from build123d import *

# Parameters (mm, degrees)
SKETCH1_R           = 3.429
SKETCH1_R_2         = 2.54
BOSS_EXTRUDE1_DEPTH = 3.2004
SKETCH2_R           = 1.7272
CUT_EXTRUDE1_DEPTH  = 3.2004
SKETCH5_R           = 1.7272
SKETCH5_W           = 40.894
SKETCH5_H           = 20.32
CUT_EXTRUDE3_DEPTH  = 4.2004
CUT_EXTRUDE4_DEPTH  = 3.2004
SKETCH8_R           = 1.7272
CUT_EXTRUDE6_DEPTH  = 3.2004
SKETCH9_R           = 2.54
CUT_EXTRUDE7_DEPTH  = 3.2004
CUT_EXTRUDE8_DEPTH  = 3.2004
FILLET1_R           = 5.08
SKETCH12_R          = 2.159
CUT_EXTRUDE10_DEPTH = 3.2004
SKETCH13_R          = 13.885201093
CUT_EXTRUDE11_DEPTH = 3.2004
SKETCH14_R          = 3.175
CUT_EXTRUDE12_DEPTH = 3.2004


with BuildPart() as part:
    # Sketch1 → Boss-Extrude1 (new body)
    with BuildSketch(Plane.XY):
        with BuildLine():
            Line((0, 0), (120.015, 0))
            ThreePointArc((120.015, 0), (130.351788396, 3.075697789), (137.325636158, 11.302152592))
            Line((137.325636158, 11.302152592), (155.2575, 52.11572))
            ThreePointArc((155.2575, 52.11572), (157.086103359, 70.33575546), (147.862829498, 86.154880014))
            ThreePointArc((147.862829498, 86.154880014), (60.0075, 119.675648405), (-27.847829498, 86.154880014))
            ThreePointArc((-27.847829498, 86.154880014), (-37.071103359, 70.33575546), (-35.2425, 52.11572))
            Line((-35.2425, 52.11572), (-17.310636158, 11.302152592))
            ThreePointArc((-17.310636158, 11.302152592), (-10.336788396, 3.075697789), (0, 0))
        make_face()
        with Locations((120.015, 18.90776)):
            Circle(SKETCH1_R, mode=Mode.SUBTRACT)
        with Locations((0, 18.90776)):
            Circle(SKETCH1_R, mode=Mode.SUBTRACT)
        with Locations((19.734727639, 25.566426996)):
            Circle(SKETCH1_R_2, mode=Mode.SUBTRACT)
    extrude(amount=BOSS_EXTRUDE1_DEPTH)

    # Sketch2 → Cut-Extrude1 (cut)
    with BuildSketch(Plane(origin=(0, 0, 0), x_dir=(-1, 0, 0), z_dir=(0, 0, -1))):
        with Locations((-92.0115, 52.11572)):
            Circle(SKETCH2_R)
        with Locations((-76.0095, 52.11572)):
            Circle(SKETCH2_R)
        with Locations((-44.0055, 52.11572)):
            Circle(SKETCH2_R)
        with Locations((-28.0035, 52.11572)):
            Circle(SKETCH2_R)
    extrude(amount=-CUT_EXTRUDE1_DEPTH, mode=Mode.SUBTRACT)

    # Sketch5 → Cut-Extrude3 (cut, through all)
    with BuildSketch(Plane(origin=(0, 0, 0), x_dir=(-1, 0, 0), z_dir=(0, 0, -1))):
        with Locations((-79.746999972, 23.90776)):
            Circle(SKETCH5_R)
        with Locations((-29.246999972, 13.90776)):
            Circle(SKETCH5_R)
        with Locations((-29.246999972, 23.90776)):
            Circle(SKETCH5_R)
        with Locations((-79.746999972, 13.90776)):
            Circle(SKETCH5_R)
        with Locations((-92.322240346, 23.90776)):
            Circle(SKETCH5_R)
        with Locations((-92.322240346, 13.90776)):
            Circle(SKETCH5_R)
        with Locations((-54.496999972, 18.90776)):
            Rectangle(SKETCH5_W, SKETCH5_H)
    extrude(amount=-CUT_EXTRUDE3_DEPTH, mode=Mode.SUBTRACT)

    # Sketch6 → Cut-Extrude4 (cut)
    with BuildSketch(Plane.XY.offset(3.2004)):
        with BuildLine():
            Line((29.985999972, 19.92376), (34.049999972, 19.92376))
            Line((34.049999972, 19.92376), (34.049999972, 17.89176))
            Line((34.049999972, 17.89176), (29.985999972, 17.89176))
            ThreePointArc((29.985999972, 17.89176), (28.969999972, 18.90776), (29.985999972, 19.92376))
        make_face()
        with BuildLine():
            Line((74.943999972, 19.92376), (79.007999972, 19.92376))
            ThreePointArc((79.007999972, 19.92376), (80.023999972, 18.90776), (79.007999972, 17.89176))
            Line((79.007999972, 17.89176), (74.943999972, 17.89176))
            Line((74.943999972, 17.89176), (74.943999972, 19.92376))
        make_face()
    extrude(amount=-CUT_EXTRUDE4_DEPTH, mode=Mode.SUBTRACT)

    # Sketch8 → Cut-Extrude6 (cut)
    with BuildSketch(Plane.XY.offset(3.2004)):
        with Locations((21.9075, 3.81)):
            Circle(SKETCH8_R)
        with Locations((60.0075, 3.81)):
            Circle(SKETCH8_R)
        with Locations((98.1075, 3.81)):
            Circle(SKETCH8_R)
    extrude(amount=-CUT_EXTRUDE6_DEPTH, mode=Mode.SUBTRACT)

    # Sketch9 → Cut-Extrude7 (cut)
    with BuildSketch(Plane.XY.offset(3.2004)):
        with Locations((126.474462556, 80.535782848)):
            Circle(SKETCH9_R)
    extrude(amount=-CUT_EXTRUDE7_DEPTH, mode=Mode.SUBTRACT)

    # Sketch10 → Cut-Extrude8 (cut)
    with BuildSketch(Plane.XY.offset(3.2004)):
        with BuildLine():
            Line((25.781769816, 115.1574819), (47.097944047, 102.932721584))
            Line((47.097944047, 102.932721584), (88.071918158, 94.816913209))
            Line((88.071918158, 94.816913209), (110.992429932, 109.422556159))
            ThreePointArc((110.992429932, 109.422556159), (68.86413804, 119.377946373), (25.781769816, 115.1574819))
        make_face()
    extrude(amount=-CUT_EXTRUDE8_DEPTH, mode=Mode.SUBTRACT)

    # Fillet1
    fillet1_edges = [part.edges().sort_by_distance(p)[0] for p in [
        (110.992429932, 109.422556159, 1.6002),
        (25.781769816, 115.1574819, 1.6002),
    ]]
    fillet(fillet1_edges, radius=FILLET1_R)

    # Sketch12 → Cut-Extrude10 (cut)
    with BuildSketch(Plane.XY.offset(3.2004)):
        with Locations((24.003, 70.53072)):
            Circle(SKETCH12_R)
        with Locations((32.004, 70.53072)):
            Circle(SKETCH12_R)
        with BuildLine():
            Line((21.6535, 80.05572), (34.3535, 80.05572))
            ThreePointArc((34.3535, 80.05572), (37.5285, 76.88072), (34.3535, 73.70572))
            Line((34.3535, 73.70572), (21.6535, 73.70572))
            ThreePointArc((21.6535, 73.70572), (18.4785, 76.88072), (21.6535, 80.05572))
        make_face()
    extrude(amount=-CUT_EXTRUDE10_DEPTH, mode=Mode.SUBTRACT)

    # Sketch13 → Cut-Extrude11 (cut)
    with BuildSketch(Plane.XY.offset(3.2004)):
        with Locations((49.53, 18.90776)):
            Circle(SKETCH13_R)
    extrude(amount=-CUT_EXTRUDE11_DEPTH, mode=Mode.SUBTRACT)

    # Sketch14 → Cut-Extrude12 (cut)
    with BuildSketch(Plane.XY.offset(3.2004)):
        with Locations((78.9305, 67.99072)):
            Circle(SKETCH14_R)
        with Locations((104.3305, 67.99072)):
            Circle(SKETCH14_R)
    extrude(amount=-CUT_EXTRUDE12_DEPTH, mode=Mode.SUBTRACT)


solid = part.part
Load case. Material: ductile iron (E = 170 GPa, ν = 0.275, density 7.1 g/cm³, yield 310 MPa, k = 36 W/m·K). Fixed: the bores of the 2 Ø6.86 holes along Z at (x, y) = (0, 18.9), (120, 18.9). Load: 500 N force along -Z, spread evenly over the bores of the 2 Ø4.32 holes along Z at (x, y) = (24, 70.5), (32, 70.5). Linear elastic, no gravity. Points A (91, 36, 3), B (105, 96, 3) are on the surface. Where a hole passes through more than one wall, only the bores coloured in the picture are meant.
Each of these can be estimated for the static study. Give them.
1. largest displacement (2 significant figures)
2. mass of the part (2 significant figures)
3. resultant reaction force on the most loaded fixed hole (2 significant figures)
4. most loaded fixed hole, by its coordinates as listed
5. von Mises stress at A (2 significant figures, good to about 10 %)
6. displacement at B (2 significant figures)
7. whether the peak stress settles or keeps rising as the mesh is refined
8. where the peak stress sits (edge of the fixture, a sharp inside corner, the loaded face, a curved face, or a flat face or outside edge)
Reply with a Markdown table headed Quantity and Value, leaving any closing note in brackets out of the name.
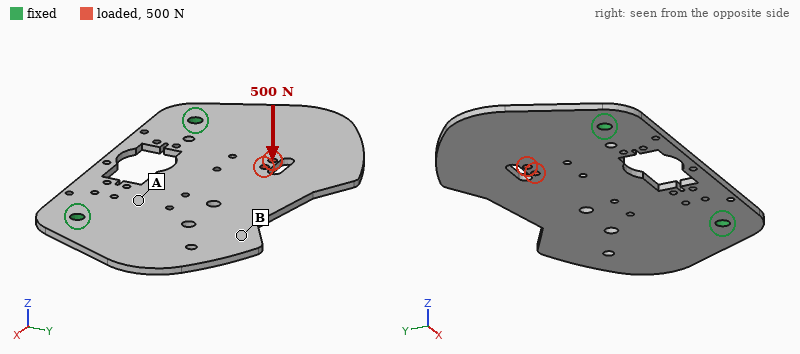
| Quantity | Value |
|---|---|
| largest displacement | 1.3 mm |
| mass of the part | 380 g |
| resultant reaction force on the most loaded fixed hole | 390 N |
| most loaded fixed hole, by its coordinates as listed | (0, 18.9) |
| von Mises stress at A | 54 MPa |
| displacement at B | 0.63 mm |
| whether the peak stress settles or keeps rising as the mesh is refined | keeps rising |
| where the peak stress sits | edge of the fixture |
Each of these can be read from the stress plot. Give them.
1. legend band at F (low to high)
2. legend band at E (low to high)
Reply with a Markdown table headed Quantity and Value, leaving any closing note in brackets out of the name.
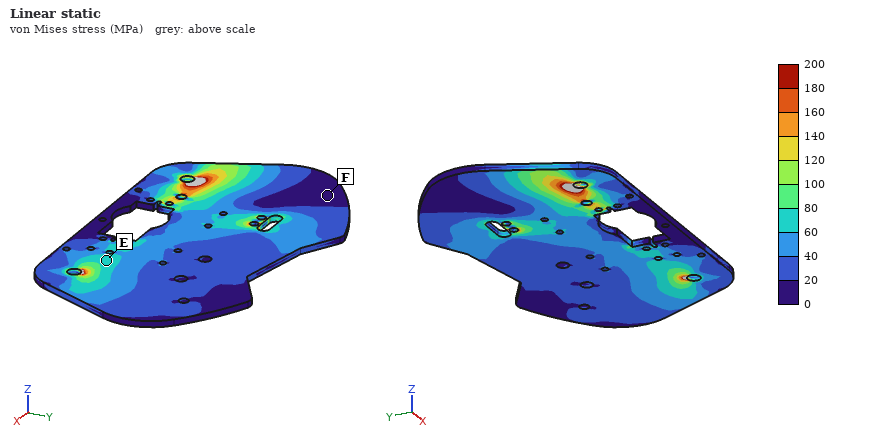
| Quantity | Value |
|---|---|
| legend band at F | 0 to 20 MPa |
| legend band at E | 60 to 80 MPa |
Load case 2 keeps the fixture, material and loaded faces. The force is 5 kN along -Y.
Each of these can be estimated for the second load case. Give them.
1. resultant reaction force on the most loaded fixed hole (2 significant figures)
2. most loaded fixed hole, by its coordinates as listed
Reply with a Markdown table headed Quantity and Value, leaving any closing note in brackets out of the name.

| Quantity | Value |
|---|---|
| resultant reaction force on the most loaded fixed hole | 4.0 kN |
| most loaded fixed hole, by its coordinates as listed | (0, 18.9) |
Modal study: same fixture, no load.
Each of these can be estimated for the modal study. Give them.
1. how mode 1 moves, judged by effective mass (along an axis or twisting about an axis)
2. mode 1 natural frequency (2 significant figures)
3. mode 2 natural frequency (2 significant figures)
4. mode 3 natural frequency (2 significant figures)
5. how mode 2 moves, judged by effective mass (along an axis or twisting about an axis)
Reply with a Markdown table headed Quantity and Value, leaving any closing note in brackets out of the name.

| Quantity | Value |
|---|---|
| how mode 1 moves, judged by effective mass | along Z |
| mode 1 natural frequency | 290 Hz |
| mode 2 natural frequency | 510 Hz |
| mode 3 natural frequency | 810 Hz |
| how mode 2 moves, judged by effective mass | twisting about Y |
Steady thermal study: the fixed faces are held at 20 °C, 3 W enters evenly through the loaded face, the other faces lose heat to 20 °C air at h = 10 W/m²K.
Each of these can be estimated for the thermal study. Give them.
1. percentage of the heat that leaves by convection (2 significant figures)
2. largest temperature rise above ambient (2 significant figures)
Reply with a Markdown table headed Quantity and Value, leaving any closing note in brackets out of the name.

| Quantity | Value |
|---|---|
| percentage of the heat that leaves by convection | 53 % |
| largest temperature rise above ambient | 23 K |
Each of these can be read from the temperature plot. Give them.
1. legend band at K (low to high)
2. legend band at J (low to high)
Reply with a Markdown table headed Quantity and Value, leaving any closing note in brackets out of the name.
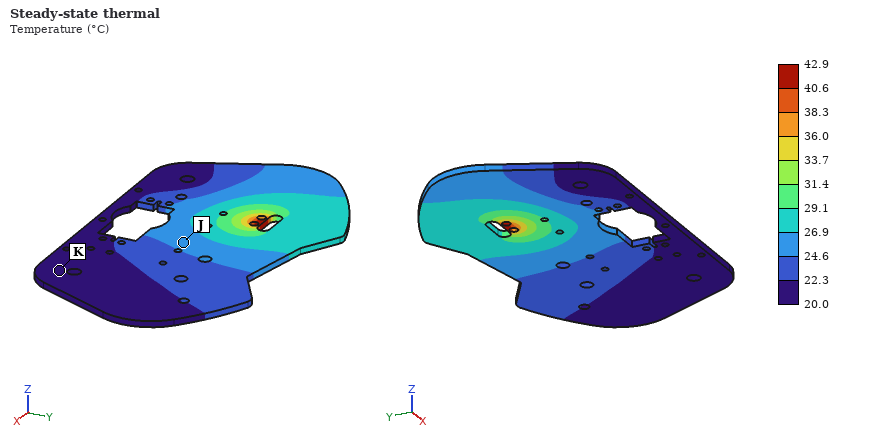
| Quantity | Value |
|---|---|
| legend band at K | 20.0 to 22.3 °C |
| legend band at J | 24.6 to 26.9 °C |
